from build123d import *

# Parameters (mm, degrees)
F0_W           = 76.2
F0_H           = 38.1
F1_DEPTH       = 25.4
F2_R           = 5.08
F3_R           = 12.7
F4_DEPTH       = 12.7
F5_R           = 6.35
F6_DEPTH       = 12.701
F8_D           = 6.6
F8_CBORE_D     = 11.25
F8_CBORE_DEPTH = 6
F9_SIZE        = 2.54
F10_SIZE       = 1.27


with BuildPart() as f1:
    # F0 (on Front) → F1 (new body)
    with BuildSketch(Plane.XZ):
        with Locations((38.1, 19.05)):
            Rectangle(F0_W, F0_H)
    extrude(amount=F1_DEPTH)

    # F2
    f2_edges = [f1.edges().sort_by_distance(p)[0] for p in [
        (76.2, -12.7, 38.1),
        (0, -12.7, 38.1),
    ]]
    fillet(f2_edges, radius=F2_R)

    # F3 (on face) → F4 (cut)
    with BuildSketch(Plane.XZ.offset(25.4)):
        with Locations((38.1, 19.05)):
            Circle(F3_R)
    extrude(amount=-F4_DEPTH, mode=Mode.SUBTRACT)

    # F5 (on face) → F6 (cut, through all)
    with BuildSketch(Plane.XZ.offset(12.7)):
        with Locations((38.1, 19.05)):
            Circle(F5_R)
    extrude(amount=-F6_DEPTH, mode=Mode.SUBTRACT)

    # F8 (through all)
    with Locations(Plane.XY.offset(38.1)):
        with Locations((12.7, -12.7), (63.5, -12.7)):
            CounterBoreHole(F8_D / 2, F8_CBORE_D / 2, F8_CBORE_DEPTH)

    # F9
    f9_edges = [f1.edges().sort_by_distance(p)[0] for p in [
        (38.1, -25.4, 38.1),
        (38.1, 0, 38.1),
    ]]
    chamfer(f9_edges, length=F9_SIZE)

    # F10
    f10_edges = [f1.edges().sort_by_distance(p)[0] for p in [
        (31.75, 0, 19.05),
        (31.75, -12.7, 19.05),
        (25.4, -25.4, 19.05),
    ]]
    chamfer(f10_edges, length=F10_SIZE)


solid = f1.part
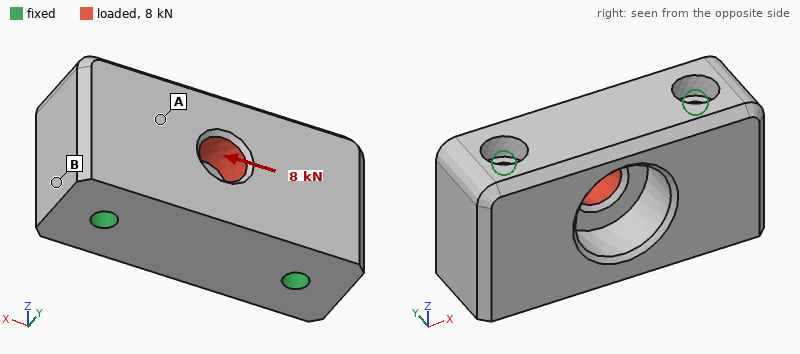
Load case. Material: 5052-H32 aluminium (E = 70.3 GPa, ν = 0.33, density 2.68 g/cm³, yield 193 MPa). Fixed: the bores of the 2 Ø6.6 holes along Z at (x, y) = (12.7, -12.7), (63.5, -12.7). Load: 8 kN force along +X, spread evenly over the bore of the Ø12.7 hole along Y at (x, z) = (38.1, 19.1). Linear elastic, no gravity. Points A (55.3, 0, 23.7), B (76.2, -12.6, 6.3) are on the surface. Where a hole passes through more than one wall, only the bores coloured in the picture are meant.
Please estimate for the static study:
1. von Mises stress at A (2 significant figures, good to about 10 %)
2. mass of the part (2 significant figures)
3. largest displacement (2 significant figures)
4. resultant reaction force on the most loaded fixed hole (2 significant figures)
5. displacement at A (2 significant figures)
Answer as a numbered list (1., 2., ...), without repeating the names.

1. 9.0 MPa
2. 160 g
3. 4.4 µm
4. 4.1 kN
5. 2.1 µm
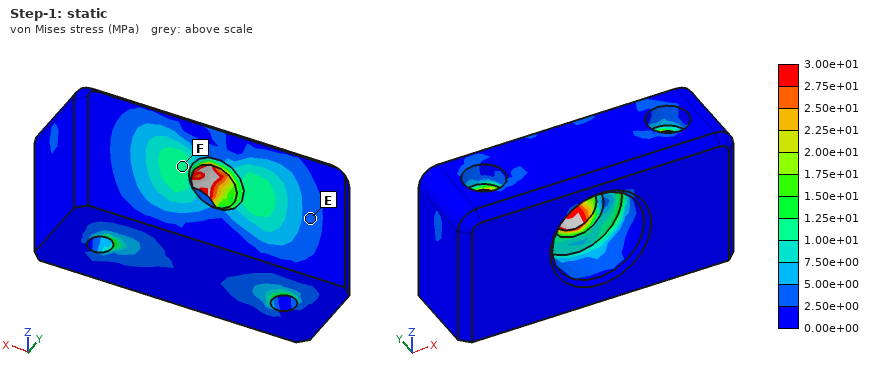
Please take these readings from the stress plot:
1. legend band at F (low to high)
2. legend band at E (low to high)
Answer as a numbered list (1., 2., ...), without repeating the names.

1. 1.00e+01 to 1.25e+01 MPa
2. 2.50e+00 to 5.00e+00 MPa
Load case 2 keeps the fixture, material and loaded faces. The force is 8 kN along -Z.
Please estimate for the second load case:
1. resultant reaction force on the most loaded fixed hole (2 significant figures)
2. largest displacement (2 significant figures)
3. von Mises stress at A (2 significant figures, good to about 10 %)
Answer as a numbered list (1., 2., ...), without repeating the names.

1. 4.0 kN
2. 9.2 µm
3. 13 MPa
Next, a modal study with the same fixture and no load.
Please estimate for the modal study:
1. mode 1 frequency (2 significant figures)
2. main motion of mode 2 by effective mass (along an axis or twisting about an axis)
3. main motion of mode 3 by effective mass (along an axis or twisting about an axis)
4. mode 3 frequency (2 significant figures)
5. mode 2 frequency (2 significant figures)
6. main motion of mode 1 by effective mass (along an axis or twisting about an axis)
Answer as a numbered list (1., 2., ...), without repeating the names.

1. 20 kHz
2. twisting about X
3. along Z
4. 28 kHz
5. 25 kHz
6. along Y
